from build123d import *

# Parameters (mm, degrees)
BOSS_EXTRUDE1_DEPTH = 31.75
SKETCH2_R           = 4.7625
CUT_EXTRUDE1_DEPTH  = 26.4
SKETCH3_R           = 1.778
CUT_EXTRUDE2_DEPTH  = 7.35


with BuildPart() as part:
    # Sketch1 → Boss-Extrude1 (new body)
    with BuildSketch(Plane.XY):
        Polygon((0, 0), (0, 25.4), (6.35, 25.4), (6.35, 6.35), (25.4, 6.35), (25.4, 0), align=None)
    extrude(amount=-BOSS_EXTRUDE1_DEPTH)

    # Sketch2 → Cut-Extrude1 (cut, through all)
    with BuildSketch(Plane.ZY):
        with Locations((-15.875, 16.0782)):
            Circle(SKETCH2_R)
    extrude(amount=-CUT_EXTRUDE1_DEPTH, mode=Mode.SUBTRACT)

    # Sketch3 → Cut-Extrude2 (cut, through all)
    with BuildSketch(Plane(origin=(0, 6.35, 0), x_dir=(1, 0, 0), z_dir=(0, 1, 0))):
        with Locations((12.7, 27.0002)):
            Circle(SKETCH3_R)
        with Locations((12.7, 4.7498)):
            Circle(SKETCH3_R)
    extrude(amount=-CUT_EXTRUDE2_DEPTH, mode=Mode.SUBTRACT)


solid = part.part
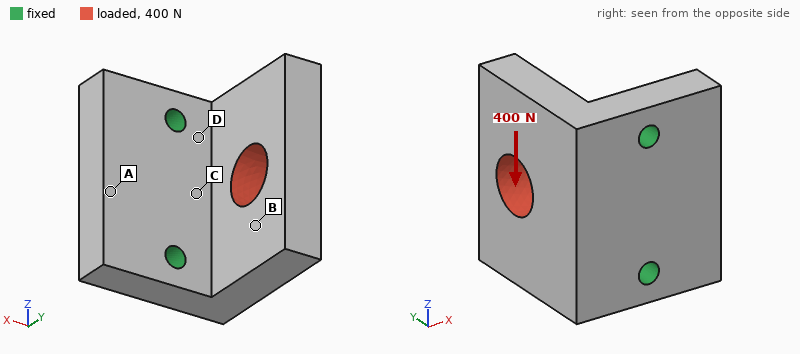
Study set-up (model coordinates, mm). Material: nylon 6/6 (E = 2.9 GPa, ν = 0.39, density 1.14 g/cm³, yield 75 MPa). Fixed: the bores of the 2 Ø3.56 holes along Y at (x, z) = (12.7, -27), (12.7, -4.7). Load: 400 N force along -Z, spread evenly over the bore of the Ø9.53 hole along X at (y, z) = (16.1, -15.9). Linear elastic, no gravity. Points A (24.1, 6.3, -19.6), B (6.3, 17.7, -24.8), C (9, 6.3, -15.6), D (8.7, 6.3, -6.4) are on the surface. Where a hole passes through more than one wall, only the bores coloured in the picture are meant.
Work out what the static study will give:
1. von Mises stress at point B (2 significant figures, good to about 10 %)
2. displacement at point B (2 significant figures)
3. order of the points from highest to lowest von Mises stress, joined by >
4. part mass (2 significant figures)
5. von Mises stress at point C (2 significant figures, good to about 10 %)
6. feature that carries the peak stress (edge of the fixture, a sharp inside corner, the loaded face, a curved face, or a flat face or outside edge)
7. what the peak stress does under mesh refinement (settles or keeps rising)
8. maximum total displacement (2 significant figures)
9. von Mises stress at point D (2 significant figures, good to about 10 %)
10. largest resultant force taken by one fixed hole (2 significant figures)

4.8 MPa
0.14 mm
D > C > B > A
9.6 g
8.4 MPa
edge of the fixture
keeps rising
0.21 mm
11 MPa
330 N
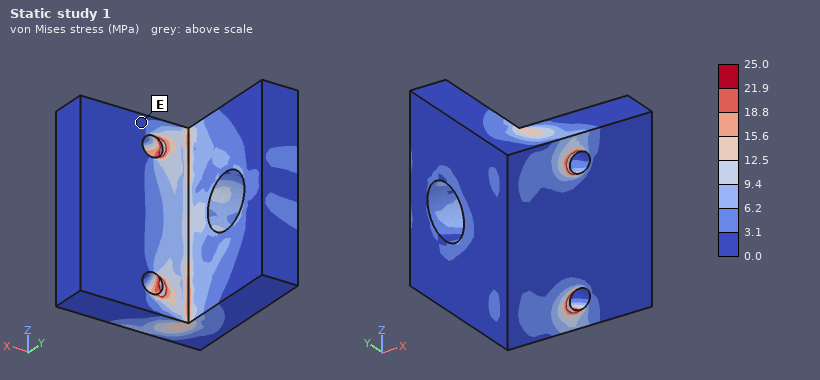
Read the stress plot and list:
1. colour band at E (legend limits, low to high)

0.0 to 3.1 MPa
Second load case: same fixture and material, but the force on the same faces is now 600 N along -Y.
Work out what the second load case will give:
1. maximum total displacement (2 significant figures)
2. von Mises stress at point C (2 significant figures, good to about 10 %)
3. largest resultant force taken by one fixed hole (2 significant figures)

0.44 mm
8.0 MPa
300 N
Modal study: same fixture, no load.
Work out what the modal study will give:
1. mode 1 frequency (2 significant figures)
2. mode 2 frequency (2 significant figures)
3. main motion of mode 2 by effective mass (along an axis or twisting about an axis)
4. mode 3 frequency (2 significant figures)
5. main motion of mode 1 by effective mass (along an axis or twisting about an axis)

2000 Hz
3700 Hz
along Z
5000 Hz
along X
